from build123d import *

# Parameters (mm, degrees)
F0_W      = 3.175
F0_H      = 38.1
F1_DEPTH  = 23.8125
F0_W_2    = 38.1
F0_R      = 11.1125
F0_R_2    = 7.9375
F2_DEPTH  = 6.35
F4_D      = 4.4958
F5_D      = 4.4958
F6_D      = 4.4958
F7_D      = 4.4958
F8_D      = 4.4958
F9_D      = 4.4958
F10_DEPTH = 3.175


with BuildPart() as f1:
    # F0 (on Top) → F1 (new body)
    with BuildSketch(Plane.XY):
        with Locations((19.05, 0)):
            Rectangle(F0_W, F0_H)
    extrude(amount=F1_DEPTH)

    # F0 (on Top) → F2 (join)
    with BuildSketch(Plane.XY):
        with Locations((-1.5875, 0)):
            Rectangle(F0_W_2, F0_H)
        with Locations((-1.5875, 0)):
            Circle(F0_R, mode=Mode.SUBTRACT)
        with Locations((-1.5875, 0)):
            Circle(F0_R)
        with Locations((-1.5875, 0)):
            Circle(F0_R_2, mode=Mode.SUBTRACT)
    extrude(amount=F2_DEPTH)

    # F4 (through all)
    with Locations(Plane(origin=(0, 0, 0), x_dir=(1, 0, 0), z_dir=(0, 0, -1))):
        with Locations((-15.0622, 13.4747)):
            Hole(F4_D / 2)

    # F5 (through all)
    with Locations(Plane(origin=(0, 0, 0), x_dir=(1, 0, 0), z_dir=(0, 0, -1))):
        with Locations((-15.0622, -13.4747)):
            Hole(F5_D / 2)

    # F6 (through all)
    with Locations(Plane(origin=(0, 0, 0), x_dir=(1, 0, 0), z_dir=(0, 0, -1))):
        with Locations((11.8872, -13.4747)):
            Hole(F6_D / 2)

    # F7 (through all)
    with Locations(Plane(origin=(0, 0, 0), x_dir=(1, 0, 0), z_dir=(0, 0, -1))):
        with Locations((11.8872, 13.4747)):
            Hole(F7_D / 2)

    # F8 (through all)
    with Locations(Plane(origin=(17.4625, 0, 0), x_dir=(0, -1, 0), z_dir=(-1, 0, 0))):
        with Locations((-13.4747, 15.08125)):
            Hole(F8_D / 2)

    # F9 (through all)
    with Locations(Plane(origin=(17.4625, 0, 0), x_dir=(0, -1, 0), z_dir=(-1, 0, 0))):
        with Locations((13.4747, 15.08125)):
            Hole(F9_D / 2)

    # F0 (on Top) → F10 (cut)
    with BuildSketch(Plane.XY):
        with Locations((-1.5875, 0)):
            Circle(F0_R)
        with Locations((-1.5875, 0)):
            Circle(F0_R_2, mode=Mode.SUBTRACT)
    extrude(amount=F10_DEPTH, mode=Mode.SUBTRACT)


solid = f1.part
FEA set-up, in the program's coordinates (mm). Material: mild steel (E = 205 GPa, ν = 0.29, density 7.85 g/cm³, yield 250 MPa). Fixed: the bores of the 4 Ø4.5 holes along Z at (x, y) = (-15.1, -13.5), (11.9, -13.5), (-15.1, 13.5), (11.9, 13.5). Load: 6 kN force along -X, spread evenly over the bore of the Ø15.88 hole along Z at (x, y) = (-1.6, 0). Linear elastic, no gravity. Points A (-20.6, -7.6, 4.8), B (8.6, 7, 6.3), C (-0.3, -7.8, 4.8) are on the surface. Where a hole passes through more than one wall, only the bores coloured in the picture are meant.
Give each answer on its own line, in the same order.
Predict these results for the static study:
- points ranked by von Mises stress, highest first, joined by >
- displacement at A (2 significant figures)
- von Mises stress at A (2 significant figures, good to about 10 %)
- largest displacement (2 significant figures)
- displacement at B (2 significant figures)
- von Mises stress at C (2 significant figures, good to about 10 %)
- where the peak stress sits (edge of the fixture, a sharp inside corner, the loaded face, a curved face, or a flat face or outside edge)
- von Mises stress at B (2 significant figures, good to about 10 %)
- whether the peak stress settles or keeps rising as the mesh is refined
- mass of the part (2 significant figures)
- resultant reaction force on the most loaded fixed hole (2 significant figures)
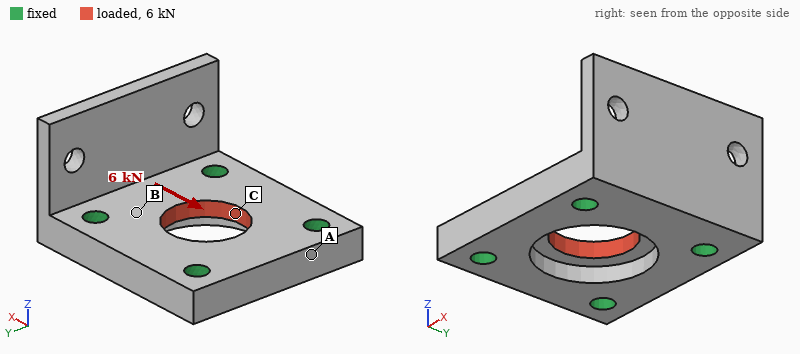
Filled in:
C > B > A
1.4 µm
10 MPa
3.9 µm
1.5 µm
67 MPa
edge of the fixture
37 MPa
keeps rising
76 g
1.6 kN
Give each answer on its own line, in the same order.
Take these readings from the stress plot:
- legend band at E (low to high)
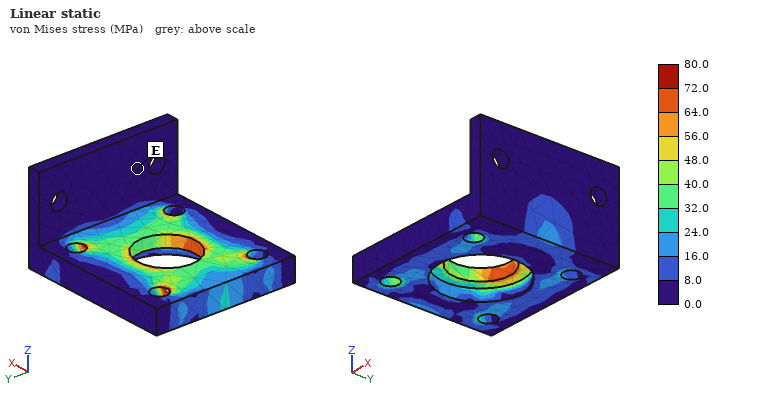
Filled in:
0.0 to 8.0 MPa
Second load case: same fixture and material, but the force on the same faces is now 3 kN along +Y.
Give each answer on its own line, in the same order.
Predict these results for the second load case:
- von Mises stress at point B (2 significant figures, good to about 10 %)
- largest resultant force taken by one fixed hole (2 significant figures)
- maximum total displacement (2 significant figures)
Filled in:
17 MPa
790 N
1.9 µm
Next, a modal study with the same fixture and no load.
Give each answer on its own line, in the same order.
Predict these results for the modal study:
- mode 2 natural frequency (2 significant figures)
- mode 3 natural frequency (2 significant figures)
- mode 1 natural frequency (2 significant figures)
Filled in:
10 kHz
19 kHz
6600 Hz
